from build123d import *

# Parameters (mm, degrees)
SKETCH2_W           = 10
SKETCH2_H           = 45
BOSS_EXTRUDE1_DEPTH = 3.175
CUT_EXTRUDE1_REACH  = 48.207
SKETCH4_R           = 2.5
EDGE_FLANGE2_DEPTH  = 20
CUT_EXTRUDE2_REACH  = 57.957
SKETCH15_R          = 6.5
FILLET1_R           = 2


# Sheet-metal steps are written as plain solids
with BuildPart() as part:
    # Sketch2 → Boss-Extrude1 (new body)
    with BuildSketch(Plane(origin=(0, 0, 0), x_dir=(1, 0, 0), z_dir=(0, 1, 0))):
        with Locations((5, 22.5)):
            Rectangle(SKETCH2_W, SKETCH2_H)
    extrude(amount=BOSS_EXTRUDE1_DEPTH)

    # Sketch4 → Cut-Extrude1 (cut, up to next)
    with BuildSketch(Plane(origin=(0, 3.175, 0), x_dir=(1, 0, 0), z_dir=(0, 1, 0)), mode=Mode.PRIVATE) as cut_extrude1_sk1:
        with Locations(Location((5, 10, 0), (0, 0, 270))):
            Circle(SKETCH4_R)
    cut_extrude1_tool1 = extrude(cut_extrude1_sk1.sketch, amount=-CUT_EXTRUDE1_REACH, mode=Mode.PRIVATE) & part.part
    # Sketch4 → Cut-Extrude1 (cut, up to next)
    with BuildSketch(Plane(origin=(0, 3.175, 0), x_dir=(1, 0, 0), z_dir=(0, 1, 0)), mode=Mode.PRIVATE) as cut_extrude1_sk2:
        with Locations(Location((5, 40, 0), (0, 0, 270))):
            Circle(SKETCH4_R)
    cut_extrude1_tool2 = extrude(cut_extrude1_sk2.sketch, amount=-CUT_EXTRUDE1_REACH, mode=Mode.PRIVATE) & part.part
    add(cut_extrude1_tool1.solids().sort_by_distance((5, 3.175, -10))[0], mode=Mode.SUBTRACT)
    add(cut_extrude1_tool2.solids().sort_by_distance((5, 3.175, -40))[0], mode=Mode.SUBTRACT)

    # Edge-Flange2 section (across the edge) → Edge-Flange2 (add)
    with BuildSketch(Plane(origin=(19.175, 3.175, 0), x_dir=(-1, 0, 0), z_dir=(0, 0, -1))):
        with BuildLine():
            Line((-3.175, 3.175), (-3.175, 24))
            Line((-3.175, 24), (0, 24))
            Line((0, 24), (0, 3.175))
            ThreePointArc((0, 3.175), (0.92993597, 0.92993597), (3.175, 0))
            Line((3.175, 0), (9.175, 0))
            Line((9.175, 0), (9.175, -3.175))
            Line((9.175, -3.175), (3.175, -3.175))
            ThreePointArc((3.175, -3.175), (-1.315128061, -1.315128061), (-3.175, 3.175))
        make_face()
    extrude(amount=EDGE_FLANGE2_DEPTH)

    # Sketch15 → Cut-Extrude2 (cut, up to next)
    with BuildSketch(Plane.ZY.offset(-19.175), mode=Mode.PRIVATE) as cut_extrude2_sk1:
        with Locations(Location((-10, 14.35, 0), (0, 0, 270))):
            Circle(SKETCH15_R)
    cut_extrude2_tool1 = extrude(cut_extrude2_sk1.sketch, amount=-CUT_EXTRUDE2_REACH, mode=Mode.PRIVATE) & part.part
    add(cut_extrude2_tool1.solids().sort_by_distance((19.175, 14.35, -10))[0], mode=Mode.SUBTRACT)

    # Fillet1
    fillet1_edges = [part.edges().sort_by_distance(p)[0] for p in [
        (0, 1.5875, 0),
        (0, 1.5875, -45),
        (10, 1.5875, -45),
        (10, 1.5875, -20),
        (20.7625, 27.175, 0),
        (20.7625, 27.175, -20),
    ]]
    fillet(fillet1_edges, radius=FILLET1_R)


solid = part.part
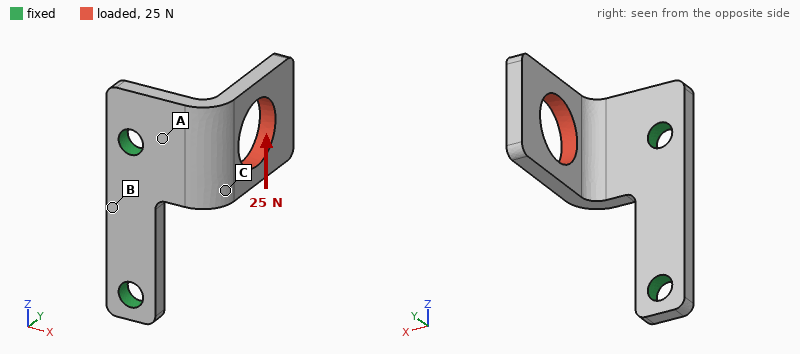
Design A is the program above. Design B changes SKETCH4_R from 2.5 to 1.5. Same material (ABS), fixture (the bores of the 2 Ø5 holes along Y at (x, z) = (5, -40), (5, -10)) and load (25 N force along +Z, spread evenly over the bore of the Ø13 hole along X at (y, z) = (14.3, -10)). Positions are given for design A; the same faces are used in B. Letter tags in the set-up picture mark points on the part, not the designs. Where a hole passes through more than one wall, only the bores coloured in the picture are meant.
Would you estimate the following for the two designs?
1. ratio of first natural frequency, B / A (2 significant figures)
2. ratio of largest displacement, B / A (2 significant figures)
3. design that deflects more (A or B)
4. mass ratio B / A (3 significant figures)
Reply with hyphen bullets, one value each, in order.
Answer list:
- 0.95
- 1.2
- B
- 1.03
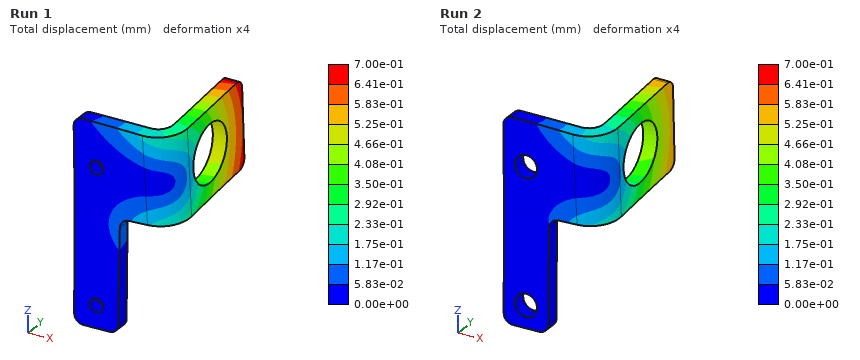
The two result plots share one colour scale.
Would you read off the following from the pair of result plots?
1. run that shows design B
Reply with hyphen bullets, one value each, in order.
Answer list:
- Run 1
